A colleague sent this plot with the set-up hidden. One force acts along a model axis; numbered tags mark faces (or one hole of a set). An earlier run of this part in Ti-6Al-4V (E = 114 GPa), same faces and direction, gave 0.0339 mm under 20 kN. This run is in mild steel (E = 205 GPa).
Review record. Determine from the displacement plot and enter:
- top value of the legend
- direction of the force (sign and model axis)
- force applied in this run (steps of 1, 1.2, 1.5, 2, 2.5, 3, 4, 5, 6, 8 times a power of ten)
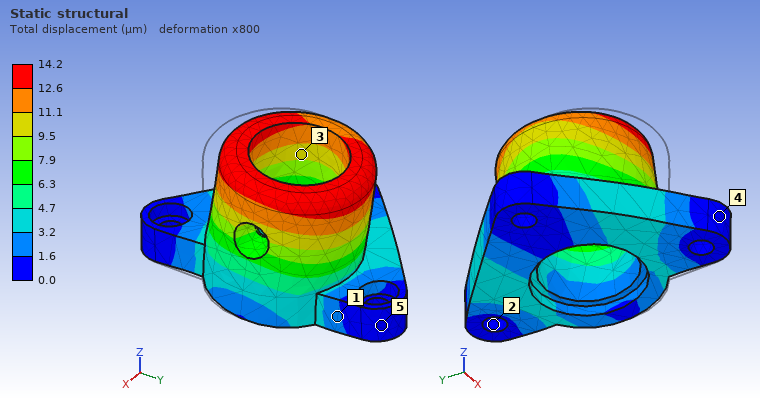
14.2 µm
+Y
15 kN
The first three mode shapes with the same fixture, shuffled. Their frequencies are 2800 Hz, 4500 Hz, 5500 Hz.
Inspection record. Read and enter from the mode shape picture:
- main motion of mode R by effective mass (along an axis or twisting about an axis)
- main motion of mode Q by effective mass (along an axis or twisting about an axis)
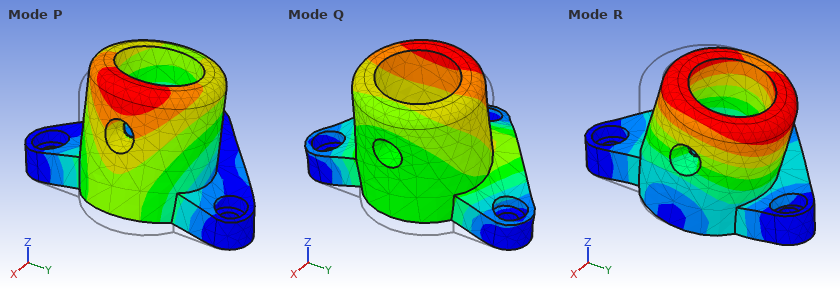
along Y
along Z
